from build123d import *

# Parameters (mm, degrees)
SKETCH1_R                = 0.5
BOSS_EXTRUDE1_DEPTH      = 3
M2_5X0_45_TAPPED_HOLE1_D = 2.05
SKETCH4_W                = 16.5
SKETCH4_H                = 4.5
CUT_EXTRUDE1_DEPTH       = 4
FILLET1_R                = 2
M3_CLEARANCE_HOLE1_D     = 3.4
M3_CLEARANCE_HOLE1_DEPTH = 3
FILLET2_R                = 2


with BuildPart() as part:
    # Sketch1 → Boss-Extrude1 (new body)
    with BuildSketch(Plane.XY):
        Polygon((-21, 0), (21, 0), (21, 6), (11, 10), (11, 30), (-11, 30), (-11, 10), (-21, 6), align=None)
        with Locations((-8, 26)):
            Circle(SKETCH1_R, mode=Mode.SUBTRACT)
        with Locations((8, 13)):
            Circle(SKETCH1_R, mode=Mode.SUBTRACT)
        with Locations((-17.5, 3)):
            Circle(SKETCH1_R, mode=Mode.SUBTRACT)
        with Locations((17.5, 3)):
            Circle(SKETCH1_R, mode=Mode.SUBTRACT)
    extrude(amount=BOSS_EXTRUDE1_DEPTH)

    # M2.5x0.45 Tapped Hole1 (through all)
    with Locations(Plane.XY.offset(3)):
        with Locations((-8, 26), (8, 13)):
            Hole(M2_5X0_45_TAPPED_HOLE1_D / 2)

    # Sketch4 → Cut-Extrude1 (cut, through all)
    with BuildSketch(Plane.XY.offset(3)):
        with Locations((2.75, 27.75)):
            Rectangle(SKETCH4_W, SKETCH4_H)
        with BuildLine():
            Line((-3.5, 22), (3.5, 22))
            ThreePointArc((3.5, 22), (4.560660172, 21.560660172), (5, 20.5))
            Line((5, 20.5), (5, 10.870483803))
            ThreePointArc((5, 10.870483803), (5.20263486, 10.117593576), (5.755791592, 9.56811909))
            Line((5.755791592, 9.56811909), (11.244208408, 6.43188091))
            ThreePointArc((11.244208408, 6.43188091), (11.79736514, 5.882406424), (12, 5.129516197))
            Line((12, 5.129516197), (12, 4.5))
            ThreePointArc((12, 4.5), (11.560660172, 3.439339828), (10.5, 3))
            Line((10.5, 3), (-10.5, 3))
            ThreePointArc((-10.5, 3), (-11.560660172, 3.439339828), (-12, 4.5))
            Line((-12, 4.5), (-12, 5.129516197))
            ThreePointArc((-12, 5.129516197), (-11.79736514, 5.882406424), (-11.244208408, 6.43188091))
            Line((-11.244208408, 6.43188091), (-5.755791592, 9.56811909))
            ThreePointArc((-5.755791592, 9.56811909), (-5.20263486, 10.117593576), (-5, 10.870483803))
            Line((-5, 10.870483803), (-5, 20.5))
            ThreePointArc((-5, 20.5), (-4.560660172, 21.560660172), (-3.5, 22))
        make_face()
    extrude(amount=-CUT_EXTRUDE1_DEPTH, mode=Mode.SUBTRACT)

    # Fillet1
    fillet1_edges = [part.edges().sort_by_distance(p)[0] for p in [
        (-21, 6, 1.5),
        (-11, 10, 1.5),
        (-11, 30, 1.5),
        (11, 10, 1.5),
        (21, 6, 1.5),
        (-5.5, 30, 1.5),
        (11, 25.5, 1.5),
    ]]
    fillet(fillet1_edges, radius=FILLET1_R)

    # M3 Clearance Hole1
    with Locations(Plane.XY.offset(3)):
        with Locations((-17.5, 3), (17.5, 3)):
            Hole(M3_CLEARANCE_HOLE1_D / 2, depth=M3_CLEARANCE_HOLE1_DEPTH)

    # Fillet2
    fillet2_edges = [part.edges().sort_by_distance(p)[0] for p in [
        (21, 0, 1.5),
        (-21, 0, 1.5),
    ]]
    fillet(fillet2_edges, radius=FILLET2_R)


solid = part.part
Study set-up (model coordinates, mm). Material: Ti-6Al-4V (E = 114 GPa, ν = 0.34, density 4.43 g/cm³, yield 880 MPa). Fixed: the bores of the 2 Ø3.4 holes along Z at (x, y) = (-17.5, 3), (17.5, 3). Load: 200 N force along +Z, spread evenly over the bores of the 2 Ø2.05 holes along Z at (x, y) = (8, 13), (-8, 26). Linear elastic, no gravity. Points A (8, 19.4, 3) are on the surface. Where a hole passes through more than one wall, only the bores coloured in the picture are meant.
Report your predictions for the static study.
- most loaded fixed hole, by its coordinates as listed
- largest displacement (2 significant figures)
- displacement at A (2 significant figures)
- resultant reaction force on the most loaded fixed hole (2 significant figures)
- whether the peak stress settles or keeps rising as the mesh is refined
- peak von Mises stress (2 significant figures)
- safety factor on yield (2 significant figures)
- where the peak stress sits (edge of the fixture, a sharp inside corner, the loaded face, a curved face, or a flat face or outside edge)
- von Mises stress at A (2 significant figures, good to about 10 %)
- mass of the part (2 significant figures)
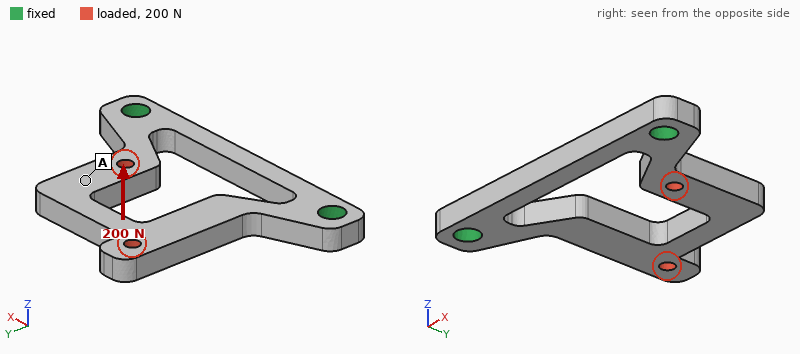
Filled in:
(17.5, 3)
0.41 mm
0.17 mm
110 N
settles
410 MPa
2.1
a curved face
35 MPa
6.1 g
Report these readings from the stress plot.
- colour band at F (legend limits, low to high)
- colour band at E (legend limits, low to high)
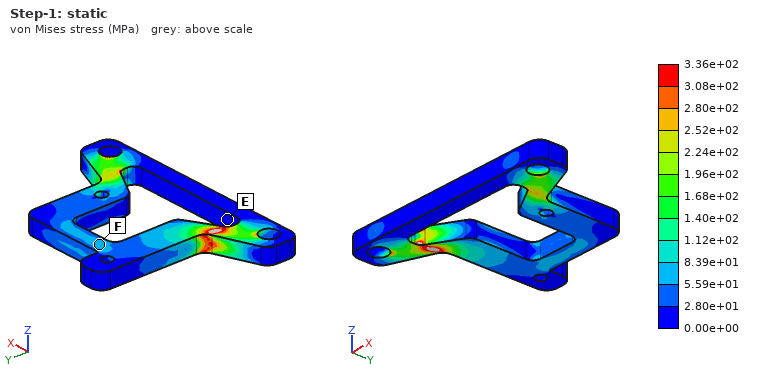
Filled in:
5.59e+01 to 8.39e+01 MPa
0.00e+00 to 2.80e+01 MPa
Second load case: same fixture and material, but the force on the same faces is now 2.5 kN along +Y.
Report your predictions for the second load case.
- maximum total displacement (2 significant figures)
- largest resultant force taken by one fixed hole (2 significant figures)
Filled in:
54 µm
1.3 kN
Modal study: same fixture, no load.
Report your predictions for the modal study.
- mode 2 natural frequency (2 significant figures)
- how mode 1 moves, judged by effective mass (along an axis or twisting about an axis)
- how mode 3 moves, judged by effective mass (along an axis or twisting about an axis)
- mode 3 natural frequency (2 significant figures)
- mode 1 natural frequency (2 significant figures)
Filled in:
7400 Hz
along Z
along X
11 kHz
2600 Hz
